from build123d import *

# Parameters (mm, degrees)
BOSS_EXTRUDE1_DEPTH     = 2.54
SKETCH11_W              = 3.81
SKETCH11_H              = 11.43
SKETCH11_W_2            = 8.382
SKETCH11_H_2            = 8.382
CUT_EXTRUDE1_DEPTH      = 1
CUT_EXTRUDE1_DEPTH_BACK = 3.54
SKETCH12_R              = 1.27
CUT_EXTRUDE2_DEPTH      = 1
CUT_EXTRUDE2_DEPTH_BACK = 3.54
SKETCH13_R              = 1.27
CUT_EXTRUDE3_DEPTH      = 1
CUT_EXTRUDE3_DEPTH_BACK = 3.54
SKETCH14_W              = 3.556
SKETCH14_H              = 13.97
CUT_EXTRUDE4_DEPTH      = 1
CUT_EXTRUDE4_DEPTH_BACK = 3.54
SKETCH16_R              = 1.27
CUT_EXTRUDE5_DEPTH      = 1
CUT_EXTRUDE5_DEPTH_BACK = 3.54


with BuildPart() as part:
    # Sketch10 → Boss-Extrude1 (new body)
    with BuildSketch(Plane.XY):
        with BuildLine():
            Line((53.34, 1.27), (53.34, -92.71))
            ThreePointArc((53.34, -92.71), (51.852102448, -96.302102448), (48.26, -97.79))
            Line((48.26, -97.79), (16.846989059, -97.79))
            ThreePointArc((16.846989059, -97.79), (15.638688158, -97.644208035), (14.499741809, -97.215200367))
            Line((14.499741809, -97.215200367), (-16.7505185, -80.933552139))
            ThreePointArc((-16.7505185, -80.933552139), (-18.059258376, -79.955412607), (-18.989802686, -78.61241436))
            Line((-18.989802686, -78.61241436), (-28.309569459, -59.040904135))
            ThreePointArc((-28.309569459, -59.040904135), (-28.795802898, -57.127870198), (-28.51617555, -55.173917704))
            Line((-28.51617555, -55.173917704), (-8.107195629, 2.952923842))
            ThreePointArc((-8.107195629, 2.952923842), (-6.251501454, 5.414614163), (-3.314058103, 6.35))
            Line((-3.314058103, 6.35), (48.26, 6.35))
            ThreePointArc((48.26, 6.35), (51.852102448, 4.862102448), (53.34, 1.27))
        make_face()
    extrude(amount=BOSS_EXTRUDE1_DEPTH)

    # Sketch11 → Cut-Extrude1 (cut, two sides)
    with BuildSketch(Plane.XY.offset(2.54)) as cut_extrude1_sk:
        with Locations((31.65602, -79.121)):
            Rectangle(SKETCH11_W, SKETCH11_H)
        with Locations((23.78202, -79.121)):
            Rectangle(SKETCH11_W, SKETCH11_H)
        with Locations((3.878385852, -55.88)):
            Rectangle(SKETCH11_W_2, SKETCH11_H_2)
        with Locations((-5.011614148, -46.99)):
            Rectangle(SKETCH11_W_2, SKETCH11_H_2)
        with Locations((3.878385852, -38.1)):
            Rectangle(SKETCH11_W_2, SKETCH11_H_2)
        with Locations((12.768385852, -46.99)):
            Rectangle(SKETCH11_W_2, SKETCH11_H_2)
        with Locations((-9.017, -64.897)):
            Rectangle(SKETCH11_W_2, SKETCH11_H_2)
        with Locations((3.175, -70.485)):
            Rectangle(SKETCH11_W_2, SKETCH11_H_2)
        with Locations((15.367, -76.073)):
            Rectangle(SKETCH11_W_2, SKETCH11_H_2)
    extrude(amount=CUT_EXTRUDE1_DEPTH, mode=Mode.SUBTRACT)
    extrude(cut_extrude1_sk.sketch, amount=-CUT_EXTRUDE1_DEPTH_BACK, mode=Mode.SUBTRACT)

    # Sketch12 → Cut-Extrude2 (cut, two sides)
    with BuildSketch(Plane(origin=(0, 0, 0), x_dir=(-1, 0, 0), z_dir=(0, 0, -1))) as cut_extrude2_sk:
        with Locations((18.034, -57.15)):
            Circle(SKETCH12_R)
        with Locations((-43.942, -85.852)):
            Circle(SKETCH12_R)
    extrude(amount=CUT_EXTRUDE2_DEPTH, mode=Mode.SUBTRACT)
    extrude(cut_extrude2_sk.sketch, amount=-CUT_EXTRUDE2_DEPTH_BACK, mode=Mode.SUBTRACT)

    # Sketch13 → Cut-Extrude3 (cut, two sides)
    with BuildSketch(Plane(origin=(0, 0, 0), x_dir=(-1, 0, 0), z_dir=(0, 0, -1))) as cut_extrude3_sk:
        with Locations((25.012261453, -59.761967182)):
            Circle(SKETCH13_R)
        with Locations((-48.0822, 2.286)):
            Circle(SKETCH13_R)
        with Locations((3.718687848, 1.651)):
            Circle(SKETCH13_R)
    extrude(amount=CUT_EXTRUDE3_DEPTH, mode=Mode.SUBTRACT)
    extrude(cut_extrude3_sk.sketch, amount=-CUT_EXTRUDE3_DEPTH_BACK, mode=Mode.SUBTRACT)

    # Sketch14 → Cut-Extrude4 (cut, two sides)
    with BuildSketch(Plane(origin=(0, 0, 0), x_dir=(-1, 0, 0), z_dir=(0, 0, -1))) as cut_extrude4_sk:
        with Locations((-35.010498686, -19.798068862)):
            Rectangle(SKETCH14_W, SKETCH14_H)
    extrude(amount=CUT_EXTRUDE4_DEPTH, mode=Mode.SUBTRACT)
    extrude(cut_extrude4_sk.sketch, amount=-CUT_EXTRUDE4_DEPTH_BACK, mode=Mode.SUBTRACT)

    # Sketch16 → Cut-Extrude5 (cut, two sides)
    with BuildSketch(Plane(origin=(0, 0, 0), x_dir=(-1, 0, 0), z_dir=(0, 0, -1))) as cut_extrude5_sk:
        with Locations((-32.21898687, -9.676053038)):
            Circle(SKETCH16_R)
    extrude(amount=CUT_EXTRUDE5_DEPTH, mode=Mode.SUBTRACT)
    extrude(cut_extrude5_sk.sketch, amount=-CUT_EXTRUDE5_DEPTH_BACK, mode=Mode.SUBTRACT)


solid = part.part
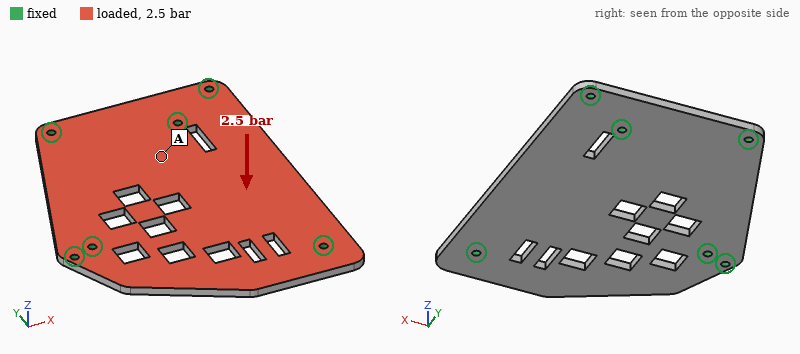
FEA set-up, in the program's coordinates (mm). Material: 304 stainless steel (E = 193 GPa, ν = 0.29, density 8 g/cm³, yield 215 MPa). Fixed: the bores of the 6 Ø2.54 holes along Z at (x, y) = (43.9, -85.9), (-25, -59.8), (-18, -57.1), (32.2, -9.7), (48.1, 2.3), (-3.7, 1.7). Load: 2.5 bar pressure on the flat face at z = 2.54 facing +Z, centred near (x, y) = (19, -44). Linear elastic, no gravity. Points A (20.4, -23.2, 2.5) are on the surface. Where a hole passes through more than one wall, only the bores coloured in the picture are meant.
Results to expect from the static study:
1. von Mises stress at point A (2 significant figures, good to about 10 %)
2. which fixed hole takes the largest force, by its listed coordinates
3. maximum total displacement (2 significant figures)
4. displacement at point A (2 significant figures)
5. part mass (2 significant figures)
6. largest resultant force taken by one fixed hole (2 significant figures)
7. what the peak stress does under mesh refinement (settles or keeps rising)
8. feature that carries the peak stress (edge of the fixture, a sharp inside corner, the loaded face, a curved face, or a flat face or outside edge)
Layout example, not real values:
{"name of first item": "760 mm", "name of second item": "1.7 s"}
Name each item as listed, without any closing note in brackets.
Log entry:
{"von Mises stress at point A": "31 MPa", "which fixed hole takes the largest force, by its listed coordinates": "(-18, -57.1)", "maximum total displacement": "0.12 mm", "displacement at point A": "0.052 mm", "part mass": "130 g", "largest resultant force taken by one fixed hole": "560 N", "what the peak stress does under mesh refinement": "keeps rising", "feature that carries the peak stress": "edge of the fixture"}
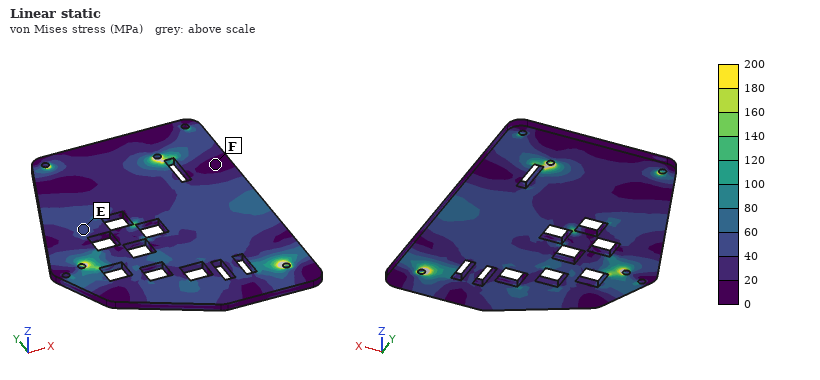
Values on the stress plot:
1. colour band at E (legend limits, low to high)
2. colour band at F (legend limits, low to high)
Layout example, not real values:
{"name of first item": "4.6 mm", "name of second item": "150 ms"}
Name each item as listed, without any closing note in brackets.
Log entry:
{"colour band at E": "40 to 60 MPa", "colour band at F": "0 to 20 MPa"}
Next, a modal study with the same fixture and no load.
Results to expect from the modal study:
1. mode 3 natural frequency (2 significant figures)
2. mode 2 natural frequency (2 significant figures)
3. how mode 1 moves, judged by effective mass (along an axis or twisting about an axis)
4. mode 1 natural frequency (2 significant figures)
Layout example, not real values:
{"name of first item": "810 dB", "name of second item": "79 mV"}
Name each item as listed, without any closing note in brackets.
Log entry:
{"mode 3 natural frequency": "3000 Hz", "mode 2 natural frequency": "2000 Hz", "how mode 1 moves, judged by effective mass": "along Z", "mode 1 natural frequency": "1900 Hz"}
